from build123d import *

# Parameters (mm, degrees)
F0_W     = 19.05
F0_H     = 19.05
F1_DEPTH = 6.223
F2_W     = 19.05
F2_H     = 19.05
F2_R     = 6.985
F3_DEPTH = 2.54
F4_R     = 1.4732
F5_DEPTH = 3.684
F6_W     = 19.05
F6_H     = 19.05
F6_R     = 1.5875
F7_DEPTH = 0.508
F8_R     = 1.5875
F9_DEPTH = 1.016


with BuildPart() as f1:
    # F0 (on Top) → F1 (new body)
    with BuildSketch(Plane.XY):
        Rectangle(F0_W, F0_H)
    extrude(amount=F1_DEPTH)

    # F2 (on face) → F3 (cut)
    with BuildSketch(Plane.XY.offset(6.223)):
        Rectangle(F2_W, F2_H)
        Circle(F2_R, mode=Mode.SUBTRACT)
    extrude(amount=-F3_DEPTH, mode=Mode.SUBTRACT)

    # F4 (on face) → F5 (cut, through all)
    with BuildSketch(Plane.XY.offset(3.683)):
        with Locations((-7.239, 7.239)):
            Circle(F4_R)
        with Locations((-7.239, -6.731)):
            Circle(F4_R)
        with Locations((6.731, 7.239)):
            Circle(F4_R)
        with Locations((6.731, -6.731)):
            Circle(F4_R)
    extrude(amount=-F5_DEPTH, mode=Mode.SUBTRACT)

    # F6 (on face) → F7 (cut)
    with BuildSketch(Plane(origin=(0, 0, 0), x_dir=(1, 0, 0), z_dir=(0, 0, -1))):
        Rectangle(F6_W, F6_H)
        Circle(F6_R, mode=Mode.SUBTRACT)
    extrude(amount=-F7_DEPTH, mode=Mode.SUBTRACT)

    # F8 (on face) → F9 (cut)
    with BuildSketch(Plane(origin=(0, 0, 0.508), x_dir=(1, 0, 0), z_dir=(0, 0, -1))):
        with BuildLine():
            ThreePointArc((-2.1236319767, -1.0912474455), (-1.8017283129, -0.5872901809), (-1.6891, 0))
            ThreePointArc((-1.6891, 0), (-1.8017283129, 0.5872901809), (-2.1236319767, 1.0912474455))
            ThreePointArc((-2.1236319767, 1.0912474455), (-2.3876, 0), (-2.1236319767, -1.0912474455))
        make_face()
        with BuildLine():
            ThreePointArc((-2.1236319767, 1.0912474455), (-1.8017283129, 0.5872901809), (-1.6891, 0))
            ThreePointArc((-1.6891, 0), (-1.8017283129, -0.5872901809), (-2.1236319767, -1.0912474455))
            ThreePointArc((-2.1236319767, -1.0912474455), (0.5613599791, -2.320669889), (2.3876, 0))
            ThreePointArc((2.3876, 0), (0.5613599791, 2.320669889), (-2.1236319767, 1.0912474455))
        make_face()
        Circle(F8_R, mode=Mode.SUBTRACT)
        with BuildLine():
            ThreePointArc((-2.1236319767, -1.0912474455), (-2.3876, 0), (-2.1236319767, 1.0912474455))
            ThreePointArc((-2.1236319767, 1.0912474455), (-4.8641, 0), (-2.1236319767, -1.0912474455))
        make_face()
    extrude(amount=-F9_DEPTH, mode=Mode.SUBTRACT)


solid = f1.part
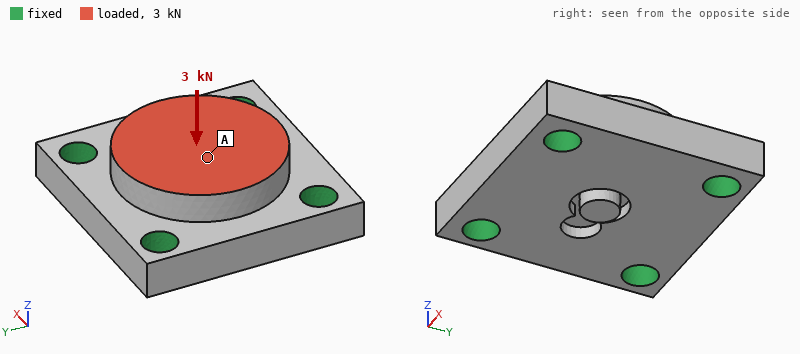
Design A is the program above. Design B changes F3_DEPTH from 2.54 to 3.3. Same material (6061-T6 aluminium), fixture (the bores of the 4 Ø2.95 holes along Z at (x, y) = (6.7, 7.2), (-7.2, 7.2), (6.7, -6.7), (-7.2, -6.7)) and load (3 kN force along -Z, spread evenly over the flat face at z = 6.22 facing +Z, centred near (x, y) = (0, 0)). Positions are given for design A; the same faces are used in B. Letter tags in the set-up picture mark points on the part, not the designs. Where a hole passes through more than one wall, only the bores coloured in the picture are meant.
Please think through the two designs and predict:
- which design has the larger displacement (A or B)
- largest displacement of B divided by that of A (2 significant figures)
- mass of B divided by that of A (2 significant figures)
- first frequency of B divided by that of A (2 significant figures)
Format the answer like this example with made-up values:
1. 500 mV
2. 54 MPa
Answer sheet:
1. B
2. 1.3
3. 0.90
4. 0.86
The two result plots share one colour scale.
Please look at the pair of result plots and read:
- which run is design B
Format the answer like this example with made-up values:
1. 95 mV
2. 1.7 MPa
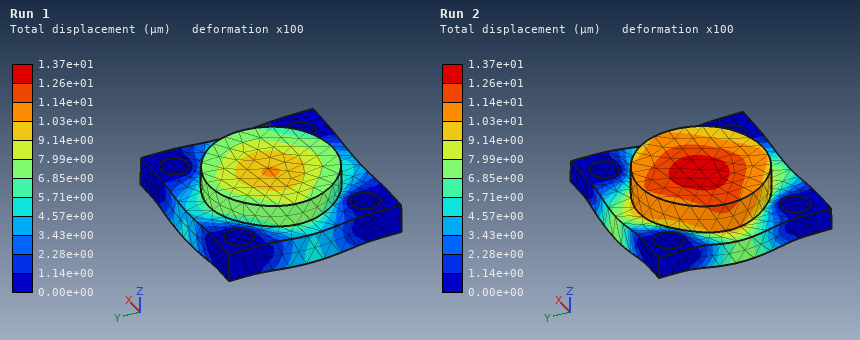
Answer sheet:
1. Run 2
